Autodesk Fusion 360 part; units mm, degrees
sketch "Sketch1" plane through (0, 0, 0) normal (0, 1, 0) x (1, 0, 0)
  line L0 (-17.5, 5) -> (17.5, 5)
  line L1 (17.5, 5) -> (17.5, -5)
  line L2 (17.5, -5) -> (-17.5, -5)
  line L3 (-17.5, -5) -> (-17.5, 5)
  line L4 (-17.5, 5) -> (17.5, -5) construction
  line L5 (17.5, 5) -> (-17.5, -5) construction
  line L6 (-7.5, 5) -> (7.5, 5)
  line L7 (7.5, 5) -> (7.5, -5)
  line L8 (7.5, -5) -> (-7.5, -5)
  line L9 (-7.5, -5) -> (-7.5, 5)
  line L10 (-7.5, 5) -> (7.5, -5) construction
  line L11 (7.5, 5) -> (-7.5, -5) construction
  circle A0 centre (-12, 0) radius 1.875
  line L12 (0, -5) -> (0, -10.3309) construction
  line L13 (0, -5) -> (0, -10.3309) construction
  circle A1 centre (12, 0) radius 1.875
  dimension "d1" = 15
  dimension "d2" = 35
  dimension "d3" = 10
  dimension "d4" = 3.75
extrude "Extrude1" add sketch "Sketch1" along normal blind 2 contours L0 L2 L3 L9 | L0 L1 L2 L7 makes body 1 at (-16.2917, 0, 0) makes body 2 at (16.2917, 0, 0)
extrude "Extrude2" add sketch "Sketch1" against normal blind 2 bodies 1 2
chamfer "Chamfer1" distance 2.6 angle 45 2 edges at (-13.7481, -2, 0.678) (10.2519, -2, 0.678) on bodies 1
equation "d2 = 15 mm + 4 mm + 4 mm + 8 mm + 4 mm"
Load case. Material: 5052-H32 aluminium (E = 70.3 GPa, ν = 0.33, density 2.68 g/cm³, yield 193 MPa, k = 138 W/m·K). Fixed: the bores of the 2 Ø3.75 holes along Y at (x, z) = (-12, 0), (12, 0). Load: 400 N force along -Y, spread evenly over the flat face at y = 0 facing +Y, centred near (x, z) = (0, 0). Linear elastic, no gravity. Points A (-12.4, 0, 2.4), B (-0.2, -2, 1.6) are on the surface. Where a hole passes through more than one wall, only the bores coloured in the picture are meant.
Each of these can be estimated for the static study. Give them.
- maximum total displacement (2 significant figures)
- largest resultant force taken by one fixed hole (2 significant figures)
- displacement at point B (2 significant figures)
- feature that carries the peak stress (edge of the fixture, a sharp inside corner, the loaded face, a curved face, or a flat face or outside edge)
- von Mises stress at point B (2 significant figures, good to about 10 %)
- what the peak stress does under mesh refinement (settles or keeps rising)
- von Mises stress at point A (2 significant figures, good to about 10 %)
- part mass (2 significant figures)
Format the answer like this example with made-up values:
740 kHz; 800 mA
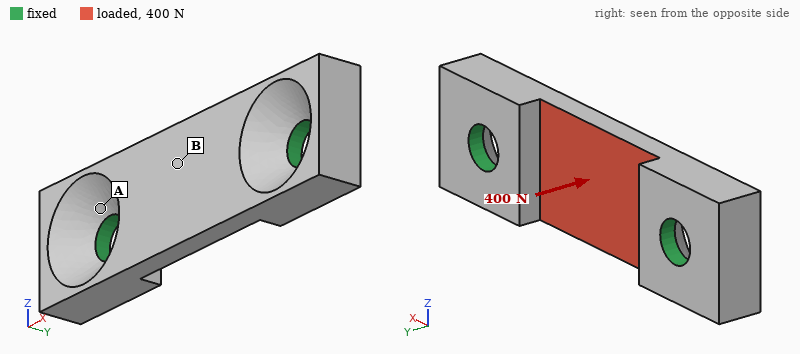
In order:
22 µm; 350 N; 20 µm; edge of the fixture; 66 MPa; keeps rising; 17 MPa; 2.4 g
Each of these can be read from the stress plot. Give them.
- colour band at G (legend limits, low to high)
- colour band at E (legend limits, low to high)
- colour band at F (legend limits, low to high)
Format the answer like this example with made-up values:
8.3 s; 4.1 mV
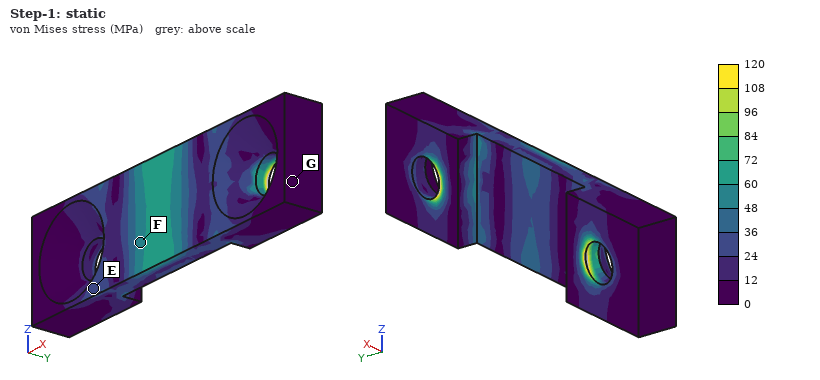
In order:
0 to 12 MPa; 24 to 36 MPa; 48 to 60 MPa
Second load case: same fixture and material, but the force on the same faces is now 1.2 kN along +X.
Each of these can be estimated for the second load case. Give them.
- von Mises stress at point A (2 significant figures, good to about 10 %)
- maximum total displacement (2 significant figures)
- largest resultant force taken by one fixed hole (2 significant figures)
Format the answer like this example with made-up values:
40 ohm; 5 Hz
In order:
63 MPa; 12 µm; 600 N
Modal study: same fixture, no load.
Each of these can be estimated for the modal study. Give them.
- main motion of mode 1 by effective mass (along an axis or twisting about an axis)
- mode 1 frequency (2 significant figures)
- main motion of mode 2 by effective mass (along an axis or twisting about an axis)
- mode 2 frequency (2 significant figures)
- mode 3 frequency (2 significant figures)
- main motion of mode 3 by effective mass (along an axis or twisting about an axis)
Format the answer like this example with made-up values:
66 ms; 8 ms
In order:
along Y; 27 kHz; along Z; 30 kHz; 40 kHz; along X
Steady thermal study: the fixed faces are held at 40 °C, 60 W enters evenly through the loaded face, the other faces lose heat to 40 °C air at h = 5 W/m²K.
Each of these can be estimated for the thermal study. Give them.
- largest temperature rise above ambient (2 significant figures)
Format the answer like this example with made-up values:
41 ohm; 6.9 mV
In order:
84 K
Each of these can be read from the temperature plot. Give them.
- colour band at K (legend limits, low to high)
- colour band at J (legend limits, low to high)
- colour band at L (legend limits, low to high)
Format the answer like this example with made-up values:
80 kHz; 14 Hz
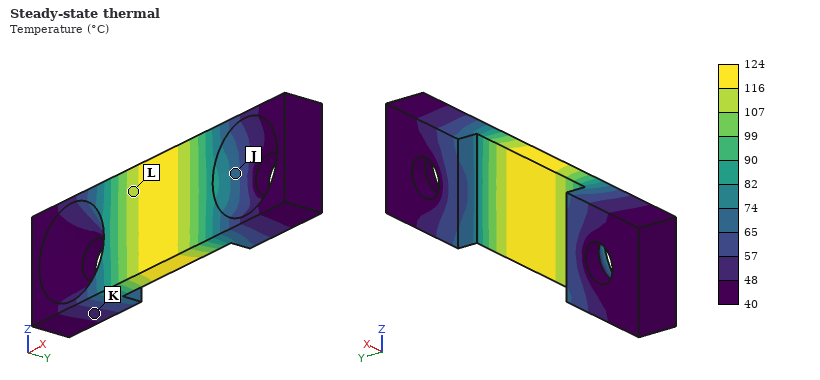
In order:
48 to 57 °C; 65 to 74 °C; 107 to 116 °C
